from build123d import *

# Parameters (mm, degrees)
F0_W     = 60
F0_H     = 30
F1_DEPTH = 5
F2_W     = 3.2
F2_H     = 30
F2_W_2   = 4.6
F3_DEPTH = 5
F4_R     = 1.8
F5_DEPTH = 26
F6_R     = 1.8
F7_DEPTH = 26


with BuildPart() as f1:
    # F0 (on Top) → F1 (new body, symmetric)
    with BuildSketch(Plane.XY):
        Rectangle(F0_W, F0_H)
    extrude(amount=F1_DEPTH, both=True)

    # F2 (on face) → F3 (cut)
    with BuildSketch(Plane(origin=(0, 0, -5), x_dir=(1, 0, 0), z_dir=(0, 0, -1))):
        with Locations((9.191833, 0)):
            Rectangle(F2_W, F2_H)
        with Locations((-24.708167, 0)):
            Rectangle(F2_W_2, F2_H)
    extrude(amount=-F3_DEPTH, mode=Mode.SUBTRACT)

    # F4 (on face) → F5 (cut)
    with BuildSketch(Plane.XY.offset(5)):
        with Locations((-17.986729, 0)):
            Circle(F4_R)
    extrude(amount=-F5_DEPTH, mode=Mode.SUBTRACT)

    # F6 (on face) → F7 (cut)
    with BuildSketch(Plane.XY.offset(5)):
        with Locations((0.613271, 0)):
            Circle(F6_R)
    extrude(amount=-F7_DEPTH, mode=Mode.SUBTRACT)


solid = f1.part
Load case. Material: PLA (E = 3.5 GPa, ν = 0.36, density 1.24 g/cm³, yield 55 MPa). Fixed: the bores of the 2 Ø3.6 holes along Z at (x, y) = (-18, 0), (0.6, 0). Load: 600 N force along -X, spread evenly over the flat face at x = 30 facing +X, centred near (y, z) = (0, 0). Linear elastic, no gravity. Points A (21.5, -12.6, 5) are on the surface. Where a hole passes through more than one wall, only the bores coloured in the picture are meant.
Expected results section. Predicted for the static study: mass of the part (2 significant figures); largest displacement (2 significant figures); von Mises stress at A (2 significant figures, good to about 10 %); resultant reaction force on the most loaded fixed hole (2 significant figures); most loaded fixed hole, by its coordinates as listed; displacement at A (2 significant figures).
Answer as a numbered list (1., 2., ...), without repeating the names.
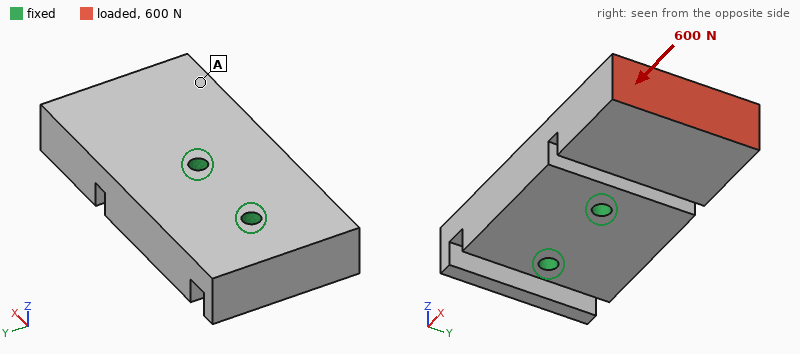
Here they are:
1. 21 g
2. 0.21 mm
3. 1.8 MPa
4. 440 N
5. (0.6, 0)
6. 0.11 mm
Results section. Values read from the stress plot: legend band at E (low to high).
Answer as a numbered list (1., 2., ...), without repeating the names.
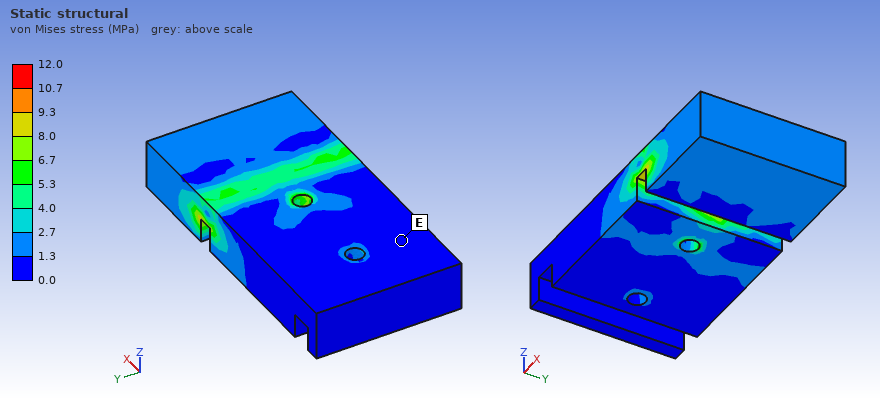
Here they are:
1. 0.0 to 1.3 MPa
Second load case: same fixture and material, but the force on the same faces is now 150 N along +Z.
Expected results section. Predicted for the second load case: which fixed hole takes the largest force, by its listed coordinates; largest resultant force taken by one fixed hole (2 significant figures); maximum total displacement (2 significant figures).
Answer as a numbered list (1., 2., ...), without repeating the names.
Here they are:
1. (0.6, 0)
2. 250 N
3. 0.58 mm
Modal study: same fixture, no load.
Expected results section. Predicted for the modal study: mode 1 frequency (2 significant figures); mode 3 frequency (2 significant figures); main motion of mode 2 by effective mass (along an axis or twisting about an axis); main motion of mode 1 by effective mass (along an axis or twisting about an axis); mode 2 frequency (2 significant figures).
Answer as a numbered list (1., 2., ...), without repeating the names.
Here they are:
1. 1500 Hz
2. 3800 Hz
3. along Y
4. along Z
5. 3300 Hz
